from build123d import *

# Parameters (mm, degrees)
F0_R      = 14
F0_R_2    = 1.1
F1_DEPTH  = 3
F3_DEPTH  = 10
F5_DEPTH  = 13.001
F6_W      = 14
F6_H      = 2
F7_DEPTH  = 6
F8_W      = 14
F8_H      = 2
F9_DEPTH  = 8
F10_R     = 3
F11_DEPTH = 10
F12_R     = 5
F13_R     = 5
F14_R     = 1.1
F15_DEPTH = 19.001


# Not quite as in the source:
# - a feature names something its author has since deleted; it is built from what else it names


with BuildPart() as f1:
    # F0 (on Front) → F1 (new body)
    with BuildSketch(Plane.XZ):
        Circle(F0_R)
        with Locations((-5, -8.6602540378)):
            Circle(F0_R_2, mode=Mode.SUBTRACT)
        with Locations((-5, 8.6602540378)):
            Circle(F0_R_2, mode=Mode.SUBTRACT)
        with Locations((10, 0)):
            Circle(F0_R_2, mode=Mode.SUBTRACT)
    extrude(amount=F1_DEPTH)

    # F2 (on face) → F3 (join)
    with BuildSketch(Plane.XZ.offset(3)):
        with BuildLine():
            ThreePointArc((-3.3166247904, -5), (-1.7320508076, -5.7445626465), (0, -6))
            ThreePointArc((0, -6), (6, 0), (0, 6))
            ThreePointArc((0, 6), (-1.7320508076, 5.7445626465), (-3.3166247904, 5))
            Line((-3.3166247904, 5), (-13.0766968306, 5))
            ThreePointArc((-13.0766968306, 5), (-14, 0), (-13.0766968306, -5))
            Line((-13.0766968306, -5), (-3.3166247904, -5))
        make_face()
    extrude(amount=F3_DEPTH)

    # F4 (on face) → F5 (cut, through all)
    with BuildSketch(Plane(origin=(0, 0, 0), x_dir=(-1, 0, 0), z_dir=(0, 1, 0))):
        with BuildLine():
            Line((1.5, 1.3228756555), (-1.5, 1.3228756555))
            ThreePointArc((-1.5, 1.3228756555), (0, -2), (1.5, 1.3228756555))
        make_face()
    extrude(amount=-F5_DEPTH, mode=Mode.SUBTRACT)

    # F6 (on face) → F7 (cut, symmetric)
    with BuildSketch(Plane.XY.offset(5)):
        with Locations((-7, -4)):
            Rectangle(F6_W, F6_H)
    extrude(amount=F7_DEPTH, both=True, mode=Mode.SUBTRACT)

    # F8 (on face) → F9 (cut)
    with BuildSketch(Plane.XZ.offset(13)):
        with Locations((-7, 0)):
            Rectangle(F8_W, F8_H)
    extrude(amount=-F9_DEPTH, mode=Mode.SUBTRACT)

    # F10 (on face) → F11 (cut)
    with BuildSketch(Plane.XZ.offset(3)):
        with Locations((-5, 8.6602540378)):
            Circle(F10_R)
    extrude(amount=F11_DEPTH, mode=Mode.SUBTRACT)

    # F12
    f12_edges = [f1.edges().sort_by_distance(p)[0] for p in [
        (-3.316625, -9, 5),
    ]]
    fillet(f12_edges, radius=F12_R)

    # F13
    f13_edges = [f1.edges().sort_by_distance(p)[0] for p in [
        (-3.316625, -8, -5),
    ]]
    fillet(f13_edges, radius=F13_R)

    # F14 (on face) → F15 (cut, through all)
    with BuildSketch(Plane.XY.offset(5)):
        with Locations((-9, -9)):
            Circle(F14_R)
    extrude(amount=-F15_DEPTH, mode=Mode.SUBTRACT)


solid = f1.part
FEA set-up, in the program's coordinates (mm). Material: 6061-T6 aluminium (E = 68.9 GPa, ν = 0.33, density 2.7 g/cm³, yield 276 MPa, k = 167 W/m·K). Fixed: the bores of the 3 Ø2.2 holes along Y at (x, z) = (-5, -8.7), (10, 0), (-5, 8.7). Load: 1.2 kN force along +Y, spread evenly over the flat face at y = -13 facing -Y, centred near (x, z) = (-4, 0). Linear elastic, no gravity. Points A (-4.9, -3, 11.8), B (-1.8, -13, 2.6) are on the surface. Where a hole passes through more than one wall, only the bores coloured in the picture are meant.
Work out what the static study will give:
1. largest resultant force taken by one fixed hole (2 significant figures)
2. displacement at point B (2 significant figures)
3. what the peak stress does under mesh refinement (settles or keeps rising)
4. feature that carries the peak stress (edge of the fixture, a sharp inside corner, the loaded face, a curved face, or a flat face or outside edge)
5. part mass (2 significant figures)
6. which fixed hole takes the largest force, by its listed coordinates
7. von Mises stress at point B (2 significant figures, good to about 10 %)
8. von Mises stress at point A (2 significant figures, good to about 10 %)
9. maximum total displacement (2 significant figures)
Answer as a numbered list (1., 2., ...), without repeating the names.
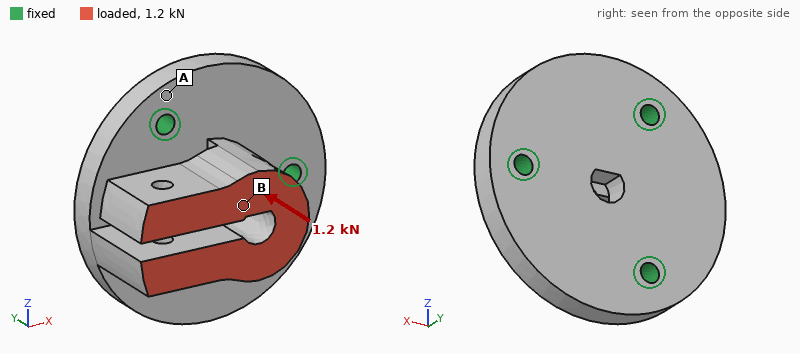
1. 580 N
2. 41 µm
3. keeps rising
4. edge of the fixture
5. 8.8 g
6. (-5, -8.7)
7. 52 MPa
8. 18 MPa
9. 92 µm
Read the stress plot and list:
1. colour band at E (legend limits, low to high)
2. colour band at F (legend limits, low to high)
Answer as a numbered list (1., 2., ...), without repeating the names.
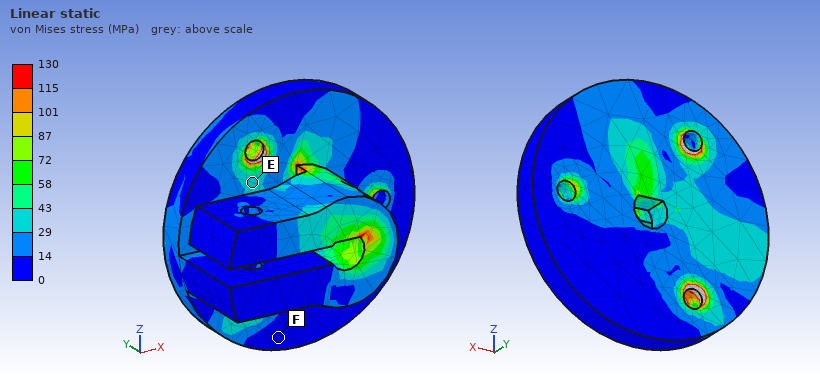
1. 29 to 43 MPa
2. 0 to 14 MPa
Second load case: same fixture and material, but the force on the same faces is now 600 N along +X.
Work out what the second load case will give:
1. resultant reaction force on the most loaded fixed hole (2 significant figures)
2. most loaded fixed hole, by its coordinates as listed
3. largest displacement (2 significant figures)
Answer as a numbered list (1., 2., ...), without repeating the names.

1. 520 N
2. (10, 0)
3. 60 µm
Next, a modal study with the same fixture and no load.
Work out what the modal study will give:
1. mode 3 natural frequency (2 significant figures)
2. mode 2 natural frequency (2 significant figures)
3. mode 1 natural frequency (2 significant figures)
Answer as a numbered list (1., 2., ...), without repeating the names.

1. 20 kHz
2. 12 kHz
3. 9500 Hz
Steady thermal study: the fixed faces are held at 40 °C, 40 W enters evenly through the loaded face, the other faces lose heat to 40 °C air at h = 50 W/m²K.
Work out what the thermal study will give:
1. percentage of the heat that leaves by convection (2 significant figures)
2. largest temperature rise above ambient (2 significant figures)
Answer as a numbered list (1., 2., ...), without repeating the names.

1. 4.8 %
2. 55 K
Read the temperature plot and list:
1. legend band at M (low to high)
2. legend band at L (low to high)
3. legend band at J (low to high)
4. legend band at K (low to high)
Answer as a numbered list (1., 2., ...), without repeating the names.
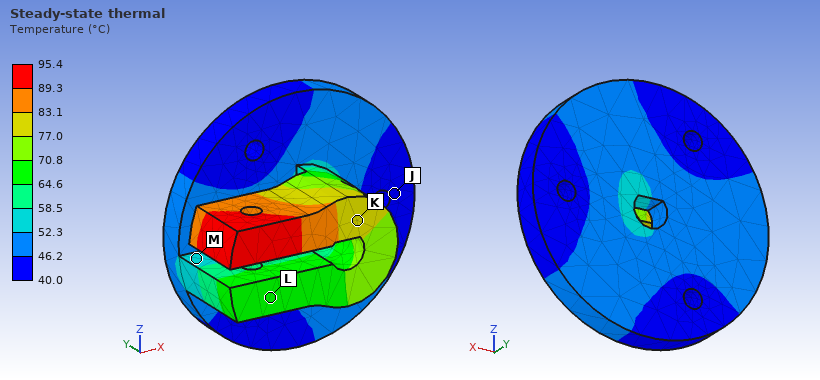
1. 52.3 to 58.5 °C
2. 64.6 to 70.8 °C
3. 40.0 to 46.2 °C
4. 77.0 to 83.1 °C
